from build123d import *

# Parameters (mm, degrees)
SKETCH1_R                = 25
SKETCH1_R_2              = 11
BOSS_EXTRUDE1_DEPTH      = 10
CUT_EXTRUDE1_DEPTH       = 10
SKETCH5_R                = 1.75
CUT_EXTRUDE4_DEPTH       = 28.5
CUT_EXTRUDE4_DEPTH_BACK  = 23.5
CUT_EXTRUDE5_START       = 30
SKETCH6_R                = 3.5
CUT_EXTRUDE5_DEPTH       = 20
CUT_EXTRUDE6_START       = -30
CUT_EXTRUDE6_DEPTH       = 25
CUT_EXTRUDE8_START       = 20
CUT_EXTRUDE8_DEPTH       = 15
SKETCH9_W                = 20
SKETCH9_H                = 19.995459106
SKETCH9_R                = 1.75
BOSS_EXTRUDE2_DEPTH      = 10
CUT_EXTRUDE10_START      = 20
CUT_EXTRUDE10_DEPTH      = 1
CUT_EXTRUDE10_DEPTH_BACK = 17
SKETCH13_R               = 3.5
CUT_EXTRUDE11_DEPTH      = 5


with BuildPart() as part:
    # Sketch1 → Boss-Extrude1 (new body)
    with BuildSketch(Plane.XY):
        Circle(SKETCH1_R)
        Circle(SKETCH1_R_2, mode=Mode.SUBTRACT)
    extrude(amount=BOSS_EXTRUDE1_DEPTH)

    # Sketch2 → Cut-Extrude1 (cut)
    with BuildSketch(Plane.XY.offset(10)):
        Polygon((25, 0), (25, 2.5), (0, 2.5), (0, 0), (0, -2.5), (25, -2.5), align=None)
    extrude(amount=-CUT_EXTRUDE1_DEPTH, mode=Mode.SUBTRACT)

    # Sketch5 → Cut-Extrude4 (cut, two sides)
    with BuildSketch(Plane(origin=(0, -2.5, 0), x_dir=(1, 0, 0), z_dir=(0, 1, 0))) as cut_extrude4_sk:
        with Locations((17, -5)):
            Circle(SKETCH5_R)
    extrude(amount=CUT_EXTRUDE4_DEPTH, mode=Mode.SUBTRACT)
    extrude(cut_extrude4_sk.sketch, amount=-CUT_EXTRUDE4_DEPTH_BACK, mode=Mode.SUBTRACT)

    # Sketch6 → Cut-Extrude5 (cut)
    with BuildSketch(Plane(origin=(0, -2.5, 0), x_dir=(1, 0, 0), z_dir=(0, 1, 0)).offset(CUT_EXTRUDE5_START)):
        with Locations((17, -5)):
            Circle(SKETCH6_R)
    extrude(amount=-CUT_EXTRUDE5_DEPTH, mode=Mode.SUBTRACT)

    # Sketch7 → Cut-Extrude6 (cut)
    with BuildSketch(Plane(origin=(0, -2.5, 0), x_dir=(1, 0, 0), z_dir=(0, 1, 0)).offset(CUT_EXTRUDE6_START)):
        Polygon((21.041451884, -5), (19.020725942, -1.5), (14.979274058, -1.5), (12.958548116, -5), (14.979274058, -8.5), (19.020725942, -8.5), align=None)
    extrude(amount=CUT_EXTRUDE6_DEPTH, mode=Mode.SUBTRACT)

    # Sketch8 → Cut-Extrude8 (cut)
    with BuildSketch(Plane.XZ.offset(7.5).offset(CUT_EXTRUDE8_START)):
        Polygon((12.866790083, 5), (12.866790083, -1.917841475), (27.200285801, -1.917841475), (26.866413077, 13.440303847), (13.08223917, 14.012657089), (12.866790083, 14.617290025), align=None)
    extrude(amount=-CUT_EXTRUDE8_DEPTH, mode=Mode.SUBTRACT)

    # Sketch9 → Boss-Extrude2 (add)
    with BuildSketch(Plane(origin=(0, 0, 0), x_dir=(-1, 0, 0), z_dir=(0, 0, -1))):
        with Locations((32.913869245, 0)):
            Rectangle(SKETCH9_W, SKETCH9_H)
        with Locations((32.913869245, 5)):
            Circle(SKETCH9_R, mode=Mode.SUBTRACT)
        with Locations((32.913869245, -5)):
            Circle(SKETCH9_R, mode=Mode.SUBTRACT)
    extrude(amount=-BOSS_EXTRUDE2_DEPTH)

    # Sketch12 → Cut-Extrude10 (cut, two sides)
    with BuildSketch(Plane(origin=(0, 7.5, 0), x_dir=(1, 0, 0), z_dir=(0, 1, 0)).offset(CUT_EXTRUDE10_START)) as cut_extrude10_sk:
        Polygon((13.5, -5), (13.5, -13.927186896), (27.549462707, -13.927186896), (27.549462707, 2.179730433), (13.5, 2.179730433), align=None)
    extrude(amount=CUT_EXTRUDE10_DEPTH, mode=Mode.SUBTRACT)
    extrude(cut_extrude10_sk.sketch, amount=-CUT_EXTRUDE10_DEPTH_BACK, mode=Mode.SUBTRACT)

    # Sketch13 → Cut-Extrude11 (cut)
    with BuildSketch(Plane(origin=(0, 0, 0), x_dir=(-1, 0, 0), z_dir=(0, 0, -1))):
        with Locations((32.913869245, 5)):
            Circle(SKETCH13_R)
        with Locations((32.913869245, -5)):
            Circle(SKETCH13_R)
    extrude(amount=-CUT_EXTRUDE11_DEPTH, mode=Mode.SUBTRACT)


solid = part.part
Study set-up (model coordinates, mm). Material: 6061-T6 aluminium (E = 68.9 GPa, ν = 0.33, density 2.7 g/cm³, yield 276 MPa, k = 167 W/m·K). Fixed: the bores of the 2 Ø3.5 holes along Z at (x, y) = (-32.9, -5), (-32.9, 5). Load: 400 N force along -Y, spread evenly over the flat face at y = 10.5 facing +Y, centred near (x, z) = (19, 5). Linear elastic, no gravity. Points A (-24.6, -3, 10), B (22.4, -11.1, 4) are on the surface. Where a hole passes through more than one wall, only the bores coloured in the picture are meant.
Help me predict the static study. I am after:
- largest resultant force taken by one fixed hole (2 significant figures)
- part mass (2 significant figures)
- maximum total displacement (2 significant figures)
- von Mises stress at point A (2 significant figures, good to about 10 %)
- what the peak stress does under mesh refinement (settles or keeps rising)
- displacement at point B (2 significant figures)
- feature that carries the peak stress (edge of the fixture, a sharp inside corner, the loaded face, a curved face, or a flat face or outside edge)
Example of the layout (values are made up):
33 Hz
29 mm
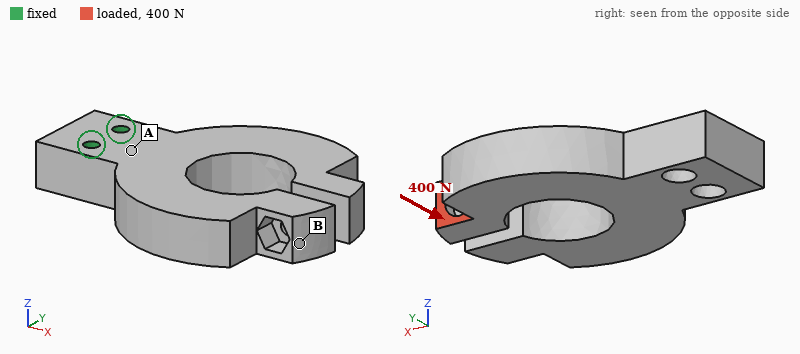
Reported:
1.7 kN
46 g
0.16 mm
27 MPa
keeps rising
0.044 mm
edge of the fixture
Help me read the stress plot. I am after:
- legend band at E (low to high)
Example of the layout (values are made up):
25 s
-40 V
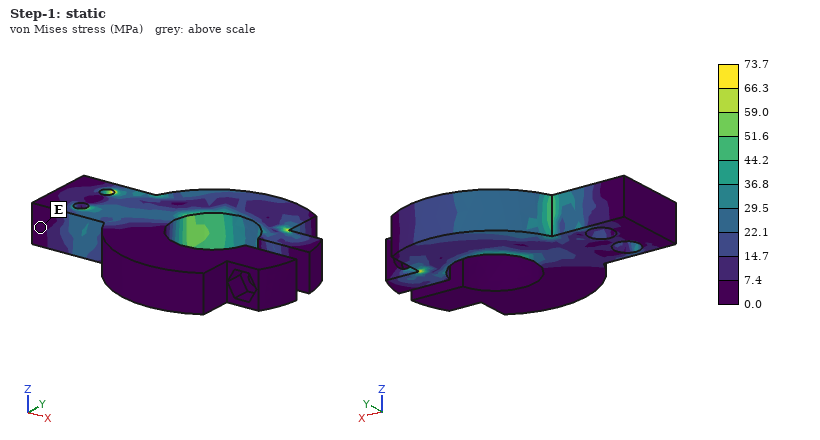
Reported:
0.0 to 7.4 MPa
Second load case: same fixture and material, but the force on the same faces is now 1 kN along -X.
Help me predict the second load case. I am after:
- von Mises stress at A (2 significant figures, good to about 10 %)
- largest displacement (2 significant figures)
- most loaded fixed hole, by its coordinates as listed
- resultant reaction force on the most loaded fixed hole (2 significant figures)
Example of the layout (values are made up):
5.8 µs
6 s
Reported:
8.9 MPa
47 µm
(-32.9, 5)
1.4 kN
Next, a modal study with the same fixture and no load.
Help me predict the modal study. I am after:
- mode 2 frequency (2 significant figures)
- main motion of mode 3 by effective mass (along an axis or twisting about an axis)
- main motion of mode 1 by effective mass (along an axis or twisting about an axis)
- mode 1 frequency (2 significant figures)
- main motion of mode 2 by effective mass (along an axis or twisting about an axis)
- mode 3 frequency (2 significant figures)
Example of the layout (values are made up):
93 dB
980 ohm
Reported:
3000 Hz
along Y
along Z
1700 Hz
along Y
3300 Hz
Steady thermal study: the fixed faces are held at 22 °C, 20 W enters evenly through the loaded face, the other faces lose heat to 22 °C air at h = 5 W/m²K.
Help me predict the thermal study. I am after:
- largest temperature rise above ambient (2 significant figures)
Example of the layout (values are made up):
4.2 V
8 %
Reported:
69 K
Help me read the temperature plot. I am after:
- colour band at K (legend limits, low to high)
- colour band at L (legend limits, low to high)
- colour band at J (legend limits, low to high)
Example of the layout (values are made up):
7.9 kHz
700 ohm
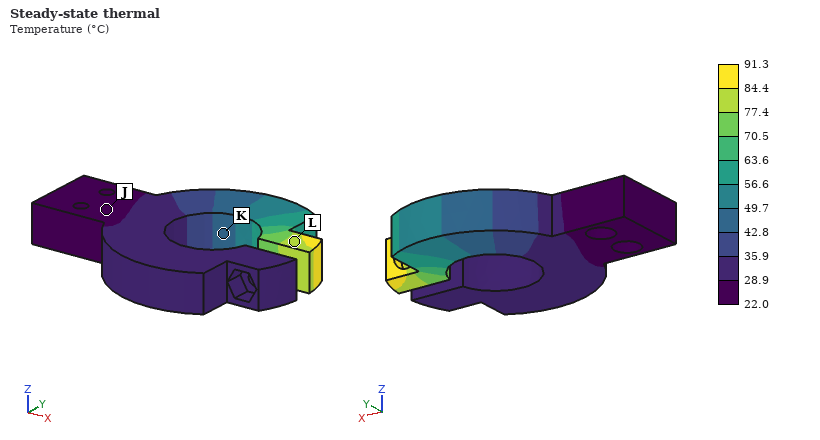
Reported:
42.8 to 49.7 °C
77.4 to 84.4 °C
22.0 to 28.9 °C
